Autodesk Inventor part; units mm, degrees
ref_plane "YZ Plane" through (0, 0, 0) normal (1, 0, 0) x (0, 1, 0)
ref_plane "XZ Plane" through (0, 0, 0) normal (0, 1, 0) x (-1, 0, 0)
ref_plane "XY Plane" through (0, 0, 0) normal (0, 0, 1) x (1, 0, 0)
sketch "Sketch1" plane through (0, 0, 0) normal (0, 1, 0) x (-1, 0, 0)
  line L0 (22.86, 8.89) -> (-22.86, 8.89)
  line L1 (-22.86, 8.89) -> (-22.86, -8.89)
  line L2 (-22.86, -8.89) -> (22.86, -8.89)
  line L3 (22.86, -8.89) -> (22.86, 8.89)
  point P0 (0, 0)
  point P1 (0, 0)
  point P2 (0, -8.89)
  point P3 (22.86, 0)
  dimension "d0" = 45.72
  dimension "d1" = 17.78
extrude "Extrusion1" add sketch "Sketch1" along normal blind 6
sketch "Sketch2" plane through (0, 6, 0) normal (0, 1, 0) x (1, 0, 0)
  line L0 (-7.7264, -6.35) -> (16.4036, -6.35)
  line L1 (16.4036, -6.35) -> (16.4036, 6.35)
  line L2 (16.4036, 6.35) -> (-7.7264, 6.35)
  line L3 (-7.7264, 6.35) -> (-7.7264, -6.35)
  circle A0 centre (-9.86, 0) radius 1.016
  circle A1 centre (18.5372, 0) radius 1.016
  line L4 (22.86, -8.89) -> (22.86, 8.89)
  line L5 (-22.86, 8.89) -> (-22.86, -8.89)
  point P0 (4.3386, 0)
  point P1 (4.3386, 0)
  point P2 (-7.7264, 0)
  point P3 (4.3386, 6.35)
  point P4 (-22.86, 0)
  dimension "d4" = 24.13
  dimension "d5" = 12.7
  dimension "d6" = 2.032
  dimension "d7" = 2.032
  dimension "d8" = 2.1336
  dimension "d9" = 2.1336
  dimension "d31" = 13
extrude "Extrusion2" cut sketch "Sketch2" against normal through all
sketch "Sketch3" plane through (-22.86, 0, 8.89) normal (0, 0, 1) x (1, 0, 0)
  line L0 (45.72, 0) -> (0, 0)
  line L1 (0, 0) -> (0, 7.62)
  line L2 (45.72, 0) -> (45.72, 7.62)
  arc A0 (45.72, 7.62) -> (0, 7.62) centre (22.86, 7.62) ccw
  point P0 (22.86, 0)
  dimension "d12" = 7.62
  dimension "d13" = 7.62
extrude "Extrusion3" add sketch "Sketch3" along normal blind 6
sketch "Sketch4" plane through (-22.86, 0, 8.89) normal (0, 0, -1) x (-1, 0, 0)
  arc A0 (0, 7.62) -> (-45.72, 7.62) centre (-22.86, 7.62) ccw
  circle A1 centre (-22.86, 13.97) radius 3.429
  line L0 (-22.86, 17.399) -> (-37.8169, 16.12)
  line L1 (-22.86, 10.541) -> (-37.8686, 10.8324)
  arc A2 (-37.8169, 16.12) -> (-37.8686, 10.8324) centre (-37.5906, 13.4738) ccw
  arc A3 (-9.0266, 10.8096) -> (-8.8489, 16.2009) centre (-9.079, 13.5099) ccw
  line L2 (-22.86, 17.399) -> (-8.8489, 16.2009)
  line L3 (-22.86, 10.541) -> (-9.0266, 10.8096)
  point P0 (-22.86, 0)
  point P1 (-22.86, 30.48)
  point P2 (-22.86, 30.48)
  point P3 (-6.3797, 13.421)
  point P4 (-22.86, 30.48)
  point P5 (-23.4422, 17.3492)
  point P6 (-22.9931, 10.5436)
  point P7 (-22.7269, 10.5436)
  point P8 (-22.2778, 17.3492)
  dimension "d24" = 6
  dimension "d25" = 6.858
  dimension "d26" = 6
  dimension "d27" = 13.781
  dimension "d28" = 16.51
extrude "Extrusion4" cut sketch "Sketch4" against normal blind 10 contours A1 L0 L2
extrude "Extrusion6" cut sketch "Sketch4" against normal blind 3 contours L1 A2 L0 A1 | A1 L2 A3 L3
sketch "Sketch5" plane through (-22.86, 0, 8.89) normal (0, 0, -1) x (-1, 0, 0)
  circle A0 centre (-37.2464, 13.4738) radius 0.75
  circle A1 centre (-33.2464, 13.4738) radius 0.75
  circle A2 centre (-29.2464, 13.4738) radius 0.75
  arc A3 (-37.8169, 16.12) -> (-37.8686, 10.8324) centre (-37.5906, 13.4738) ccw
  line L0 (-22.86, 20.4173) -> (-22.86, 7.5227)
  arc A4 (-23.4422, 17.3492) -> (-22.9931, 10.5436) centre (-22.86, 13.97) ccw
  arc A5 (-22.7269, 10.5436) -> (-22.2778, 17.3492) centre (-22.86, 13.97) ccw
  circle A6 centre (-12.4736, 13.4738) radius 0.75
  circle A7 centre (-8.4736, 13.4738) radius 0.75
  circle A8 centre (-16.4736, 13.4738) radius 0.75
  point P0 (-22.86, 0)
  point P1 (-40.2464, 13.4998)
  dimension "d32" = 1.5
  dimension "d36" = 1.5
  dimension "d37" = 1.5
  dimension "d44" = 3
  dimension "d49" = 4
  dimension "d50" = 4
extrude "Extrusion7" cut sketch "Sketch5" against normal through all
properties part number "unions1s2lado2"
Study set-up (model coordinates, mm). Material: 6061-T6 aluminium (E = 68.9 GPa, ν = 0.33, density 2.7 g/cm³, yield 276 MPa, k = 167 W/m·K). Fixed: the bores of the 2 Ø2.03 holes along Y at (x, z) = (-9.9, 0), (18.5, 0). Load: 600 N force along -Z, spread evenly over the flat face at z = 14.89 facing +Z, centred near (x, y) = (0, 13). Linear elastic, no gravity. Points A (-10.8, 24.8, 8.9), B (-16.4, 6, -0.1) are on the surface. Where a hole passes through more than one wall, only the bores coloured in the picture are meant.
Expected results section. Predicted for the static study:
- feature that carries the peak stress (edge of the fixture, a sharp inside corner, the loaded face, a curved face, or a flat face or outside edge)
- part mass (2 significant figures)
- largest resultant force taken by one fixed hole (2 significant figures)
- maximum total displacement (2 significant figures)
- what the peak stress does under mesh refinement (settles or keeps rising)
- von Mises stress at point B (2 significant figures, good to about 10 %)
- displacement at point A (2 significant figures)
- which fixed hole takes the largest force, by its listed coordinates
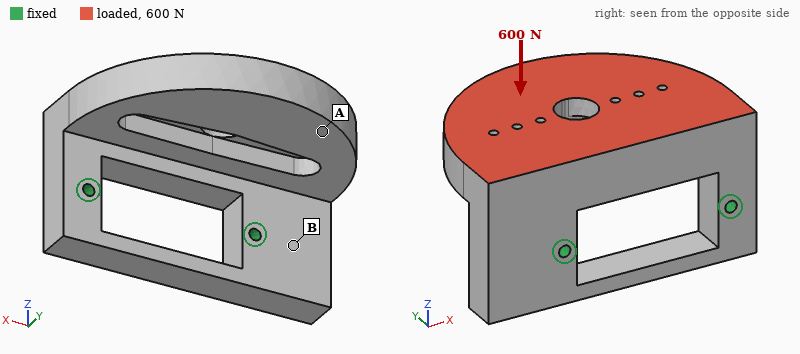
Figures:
edge of the fixture
25 g
390 N
0.13 mm
keeps rising
23 MPa
0.090 mm
(-9.9, 0)
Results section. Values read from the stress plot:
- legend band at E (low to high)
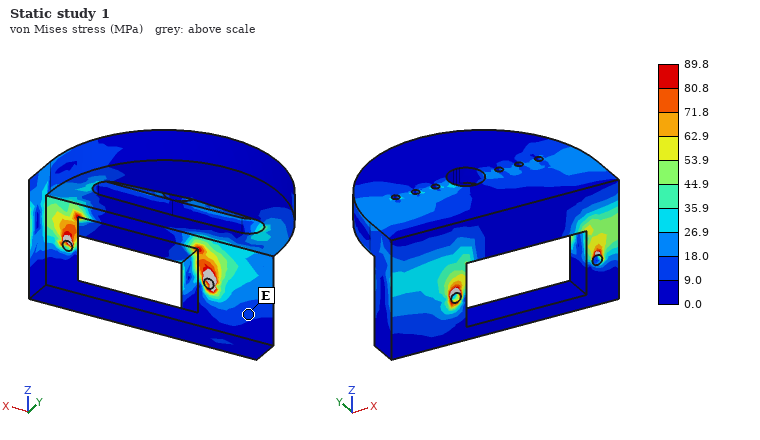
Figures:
9.0 to 18.0 MPa
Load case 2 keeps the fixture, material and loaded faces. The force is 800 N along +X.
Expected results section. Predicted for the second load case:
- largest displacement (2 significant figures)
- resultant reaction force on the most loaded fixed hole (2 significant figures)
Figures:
26 µm
580 N
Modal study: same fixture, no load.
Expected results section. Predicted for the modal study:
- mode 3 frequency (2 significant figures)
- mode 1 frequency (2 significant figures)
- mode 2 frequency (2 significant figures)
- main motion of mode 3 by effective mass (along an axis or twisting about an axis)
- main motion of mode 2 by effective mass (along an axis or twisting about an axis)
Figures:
9000 Hz
3200 Hz
6800 Hz
along Y
along X
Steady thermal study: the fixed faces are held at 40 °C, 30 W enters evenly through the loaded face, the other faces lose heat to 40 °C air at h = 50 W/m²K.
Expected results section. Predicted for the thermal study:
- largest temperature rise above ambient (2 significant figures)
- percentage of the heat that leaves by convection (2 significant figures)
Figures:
26 K
9.1 %
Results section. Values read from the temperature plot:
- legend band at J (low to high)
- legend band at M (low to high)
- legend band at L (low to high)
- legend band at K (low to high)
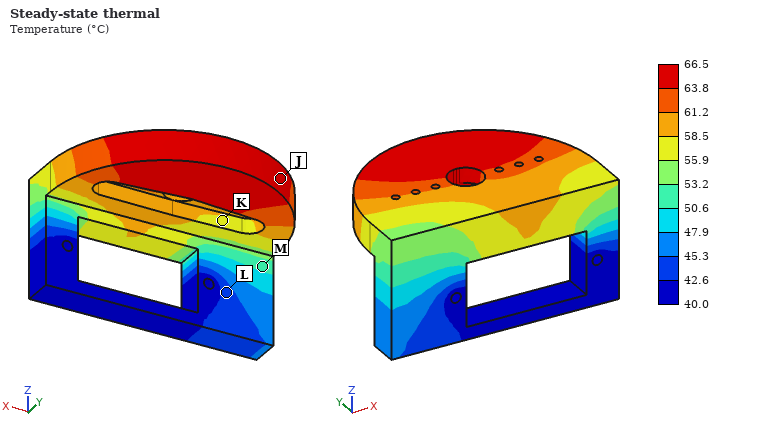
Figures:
63.8 to 66.5 °C
50.6 to 53.2 °C
42.6 to 45.3 °C
55.9 to 58.5 °C
